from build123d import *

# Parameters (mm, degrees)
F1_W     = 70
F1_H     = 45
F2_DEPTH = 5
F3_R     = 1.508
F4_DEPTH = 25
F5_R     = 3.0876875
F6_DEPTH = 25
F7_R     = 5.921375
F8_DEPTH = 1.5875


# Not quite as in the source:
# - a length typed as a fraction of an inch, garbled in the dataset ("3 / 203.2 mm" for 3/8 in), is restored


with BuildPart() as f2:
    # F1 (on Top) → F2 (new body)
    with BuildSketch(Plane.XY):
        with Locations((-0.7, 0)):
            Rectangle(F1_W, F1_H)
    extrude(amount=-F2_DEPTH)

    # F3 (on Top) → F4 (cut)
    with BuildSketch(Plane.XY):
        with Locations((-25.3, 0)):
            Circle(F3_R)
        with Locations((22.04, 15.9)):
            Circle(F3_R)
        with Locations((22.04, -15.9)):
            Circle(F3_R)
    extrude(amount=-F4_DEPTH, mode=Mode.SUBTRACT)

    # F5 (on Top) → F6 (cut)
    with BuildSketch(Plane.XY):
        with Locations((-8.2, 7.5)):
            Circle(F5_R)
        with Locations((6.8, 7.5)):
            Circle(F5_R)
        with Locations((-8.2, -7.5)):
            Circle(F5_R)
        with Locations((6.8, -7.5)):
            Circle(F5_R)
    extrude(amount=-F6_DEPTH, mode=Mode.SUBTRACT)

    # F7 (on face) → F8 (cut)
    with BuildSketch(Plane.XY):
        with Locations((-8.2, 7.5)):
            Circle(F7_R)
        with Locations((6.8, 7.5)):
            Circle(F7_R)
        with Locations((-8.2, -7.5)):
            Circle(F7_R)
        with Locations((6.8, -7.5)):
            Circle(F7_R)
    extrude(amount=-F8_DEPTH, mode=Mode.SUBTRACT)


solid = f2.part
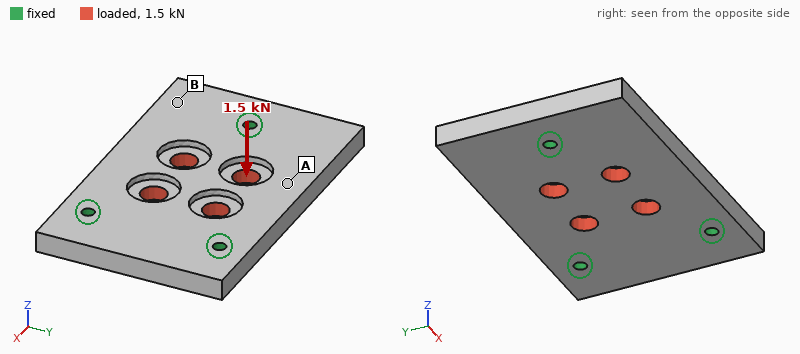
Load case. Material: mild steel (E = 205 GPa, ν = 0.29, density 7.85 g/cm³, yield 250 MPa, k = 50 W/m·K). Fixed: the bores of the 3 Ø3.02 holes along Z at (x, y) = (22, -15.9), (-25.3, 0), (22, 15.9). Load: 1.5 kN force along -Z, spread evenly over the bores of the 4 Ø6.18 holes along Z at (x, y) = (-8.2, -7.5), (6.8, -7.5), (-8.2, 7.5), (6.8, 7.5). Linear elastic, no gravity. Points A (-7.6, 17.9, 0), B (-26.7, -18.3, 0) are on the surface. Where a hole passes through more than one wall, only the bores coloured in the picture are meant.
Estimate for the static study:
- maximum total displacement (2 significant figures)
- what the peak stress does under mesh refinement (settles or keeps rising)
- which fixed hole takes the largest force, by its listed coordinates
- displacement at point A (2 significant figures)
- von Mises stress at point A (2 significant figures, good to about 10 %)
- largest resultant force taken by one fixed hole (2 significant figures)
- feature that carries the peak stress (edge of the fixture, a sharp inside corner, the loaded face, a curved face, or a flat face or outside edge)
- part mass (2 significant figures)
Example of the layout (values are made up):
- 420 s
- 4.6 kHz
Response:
- 16 µm
- keeps rising
- (-25.3, 0)
- 11 µm
- 35 MPa
- 700 N
- edge of the fixture
- 110 g
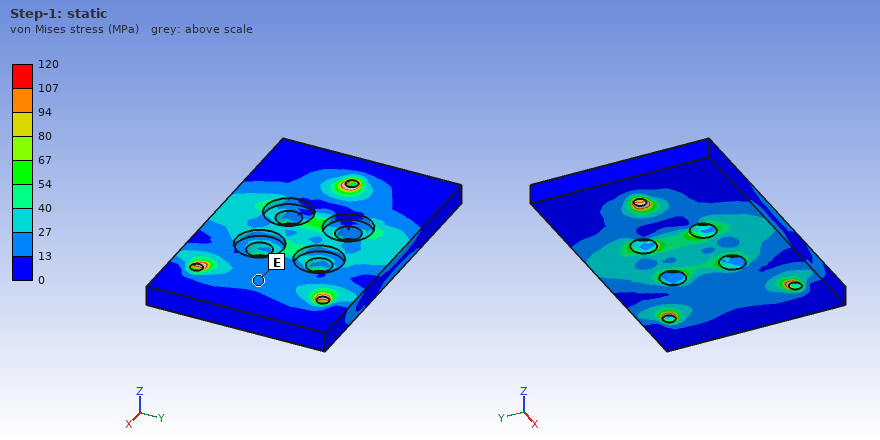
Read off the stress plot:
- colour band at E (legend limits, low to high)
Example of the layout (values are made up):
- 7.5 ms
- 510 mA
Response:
- 13 to 27 MPa
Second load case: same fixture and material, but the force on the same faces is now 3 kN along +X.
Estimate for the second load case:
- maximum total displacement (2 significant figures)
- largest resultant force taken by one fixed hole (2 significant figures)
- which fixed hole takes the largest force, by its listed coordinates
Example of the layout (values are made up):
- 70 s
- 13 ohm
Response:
- 1.7 µm
- 1.2 kN
- (-25.3, 0)
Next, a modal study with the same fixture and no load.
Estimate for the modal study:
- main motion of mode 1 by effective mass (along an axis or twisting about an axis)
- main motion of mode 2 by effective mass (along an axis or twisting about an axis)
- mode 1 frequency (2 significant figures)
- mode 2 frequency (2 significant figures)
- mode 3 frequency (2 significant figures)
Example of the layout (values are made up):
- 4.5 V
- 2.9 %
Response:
- twisting about X
- along Z
- 6200 Hz
- 7600 Hz
- 10 kHz
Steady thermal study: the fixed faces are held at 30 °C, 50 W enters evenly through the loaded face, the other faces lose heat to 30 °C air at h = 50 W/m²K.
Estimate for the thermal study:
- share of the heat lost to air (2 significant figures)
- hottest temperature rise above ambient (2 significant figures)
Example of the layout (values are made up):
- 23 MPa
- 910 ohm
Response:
- 19 %
- 63 K
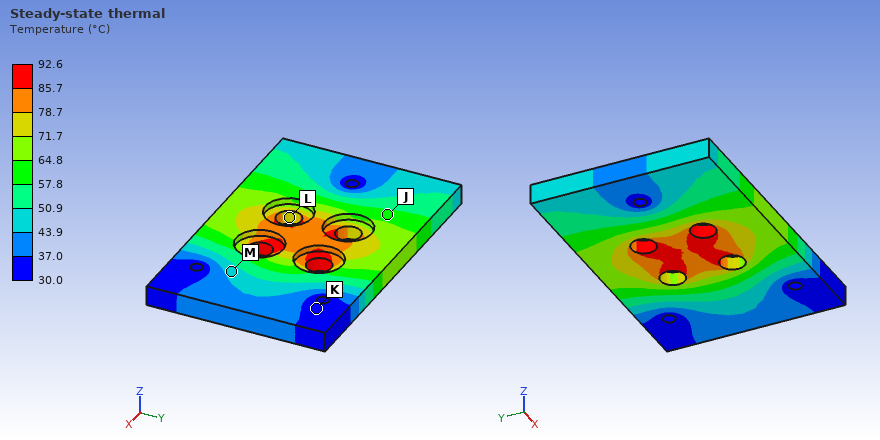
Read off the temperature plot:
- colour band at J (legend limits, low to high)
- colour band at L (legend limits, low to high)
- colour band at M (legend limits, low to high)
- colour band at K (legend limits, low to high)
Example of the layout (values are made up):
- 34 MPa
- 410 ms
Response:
- 57.8 to 64.8 °C
- 71.7 to 78.7 °C
- 43.9 to 50.9 °C
- 30.0 to 37.0 °C
